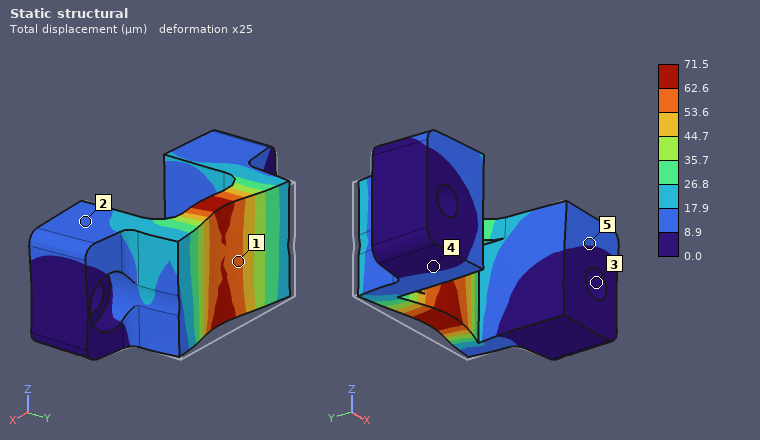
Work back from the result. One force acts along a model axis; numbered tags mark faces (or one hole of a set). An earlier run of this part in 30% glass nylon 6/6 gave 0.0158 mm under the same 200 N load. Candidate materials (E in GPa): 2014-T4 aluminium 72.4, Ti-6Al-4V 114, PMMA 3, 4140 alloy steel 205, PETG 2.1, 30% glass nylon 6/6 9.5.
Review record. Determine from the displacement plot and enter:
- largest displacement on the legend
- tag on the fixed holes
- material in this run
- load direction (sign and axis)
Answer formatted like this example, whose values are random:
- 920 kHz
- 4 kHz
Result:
- 71.5 µm
- 3
- PETG
- -Y
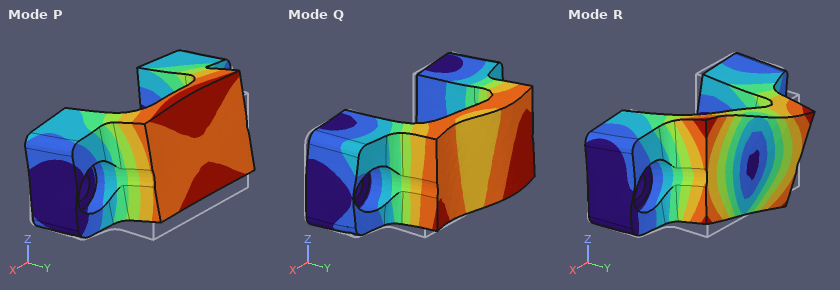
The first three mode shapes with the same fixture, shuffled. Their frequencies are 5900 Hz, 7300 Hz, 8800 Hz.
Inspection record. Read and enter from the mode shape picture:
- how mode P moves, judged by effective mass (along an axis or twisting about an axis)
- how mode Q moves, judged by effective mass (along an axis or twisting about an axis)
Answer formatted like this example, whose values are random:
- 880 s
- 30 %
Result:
- along Z
- along X
